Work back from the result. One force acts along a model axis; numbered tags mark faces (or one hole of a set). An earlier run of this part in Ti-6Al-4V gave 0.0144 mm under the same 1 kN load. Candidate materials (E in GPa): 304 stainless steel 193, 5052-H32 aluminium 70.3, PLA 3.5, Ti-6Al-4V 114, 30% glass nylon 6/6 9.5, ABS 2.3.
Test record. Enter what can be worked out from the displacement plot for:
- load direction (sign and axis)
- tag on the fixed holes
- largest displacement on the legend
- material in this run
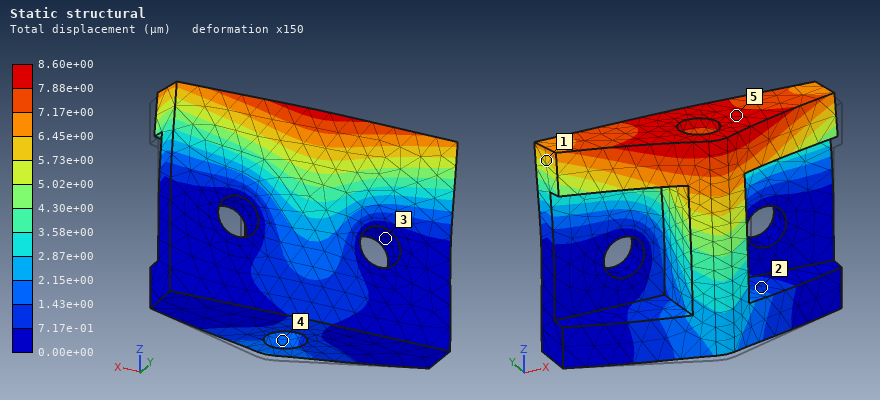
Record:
+Y
3
8.60e+00 µm
304 stainless steel
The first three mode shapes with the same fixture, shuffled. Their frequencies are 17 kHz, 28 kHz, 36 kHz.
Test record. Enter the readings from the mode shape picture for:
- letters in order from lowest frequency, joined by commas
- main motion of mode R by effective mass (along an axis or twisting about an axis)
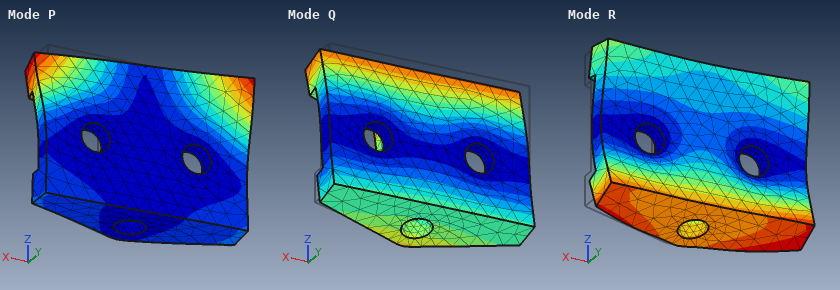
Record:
Q, P, R
along Y
